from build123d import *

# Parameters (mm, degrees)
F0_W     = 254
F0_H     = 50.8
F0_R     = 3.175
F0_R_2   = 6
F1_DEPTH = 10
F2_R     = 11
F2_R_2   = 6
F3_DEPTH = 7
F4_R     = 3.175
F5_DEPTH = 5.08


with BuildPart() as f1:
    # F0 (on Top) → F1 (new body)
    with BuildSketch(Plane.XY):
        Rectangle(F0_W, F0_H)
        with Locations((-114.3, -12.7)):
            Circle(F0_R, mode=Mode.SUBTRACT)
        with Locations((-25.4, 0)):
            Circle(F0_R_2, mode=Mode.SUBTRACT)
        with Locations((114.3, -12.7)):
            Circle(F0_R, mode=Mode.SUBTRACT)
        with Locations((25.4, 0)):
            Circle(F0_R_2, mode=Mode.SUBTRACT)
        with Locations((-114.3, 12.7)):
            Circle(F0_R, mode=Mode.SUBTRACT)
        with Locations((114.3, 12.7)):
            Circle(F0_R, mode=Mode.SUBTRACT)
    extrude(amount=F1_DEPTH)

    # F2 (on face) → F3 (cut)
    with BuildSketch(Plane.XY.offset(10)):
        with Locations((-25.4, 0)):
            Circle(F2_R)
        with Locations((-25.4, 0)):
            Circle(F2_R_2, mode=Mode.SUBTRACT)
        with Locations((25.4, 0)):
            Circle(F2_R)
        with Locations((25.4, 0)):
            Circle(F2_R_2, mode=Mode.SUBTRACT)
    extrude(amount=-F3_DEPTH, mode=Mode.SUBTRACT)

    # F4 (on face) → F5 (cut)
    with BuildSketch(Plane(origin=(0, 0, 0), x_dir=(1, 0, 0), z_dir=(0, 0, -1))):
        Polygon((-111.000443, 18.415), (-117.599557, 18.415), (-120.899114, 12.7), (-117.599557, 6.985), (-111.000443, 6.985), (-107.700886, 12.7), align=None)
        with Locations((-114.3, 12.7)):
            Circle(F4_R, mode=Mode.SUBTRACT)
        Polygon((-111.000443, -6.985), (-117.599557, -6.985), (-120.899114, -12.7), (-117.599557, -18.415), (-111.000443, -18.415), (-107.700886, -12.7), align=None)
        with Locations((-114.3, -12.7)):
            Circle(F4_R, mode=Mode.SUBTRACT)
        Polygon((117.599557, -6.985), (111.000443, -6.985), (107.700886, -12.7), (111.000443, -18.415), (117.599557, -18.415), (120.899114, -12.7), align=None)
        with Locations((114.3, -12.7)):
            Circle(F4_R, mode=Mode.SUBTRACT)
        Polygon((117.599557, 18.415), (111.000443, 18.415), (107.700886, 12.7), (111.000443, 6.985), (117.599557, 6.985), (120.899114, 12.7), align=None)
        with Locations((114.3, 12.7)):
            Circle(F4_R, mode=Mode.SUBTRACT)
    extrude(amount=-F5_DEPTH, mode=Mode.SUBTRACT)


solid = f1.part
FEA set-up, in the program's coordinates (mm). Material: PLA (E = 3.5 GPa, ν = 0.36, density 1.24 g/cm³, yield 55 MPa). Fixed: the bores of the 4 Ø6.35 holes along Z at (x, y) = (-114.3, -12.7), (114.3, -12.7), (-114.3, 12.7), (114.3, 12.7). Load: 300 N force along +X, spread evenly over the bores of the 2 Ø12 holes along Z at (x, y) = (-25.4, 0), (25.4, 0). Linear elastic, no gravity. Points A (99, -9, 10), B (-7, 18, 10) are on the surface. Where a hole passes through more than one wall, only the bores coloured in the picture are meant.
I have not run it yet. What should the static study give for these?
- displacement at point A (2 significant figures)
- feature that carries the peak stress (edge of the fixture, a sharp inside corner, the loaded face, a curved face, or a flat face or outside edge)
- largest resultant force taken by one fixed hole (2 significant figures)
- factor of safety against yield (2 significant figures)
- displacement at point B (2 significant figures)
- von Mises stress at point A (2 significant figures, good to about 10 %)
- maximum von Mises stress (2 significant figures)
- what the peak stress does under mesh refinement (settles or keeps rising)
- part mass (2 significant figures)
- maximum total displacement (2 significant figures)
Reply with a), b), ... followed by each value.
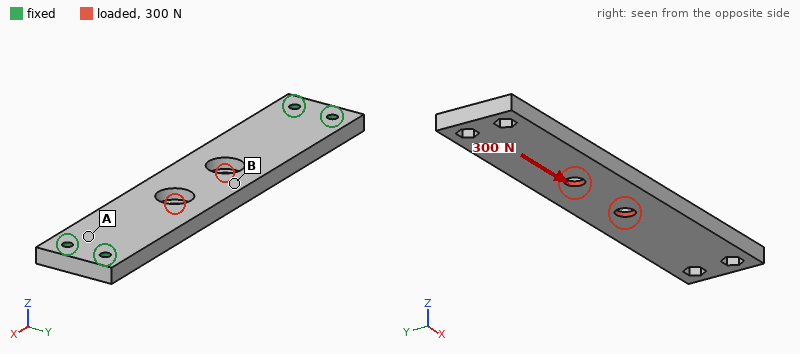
a) 2.5 µm
b) the loaded face
c) 76 N
d) 22
e) 8.4 µm
f) 0.53 MPa
g) 2.5 MPa
h) settles
i) 150 g
j) 16 µm
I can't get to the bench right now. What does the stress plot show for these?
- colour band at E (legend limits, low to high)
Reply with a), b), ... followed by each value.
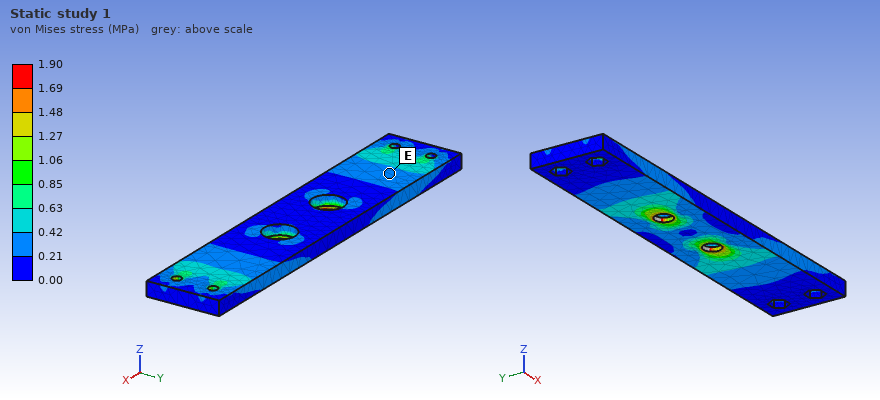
a) 0.21 to 0.42 MPa
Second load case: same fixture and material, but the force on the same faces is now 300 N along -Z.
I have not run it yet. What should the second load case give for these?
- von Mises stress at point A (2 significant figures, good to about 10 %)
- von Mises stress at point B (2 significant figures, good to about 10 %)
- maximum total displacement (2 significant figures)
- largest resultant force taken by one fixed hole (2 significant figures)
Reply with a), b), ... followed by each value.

a) 6.6 MPa
b) 6.8 MPa
c) 1.6 mm
d) 210 N
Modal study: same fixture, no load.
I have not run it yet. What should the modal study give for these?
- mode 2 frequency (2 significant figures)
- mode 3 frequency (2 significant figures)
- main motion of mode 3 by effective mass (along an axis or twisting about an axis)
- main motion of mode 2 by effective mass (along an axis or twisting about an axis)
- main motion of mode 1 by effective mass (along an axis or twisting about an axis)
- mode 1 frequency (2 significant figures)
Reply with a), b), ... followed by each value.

a) 760 Hz
b) 830 Hz
c) twisting about X
d) twisting about Y
e) along Z
f) 280 Hz
